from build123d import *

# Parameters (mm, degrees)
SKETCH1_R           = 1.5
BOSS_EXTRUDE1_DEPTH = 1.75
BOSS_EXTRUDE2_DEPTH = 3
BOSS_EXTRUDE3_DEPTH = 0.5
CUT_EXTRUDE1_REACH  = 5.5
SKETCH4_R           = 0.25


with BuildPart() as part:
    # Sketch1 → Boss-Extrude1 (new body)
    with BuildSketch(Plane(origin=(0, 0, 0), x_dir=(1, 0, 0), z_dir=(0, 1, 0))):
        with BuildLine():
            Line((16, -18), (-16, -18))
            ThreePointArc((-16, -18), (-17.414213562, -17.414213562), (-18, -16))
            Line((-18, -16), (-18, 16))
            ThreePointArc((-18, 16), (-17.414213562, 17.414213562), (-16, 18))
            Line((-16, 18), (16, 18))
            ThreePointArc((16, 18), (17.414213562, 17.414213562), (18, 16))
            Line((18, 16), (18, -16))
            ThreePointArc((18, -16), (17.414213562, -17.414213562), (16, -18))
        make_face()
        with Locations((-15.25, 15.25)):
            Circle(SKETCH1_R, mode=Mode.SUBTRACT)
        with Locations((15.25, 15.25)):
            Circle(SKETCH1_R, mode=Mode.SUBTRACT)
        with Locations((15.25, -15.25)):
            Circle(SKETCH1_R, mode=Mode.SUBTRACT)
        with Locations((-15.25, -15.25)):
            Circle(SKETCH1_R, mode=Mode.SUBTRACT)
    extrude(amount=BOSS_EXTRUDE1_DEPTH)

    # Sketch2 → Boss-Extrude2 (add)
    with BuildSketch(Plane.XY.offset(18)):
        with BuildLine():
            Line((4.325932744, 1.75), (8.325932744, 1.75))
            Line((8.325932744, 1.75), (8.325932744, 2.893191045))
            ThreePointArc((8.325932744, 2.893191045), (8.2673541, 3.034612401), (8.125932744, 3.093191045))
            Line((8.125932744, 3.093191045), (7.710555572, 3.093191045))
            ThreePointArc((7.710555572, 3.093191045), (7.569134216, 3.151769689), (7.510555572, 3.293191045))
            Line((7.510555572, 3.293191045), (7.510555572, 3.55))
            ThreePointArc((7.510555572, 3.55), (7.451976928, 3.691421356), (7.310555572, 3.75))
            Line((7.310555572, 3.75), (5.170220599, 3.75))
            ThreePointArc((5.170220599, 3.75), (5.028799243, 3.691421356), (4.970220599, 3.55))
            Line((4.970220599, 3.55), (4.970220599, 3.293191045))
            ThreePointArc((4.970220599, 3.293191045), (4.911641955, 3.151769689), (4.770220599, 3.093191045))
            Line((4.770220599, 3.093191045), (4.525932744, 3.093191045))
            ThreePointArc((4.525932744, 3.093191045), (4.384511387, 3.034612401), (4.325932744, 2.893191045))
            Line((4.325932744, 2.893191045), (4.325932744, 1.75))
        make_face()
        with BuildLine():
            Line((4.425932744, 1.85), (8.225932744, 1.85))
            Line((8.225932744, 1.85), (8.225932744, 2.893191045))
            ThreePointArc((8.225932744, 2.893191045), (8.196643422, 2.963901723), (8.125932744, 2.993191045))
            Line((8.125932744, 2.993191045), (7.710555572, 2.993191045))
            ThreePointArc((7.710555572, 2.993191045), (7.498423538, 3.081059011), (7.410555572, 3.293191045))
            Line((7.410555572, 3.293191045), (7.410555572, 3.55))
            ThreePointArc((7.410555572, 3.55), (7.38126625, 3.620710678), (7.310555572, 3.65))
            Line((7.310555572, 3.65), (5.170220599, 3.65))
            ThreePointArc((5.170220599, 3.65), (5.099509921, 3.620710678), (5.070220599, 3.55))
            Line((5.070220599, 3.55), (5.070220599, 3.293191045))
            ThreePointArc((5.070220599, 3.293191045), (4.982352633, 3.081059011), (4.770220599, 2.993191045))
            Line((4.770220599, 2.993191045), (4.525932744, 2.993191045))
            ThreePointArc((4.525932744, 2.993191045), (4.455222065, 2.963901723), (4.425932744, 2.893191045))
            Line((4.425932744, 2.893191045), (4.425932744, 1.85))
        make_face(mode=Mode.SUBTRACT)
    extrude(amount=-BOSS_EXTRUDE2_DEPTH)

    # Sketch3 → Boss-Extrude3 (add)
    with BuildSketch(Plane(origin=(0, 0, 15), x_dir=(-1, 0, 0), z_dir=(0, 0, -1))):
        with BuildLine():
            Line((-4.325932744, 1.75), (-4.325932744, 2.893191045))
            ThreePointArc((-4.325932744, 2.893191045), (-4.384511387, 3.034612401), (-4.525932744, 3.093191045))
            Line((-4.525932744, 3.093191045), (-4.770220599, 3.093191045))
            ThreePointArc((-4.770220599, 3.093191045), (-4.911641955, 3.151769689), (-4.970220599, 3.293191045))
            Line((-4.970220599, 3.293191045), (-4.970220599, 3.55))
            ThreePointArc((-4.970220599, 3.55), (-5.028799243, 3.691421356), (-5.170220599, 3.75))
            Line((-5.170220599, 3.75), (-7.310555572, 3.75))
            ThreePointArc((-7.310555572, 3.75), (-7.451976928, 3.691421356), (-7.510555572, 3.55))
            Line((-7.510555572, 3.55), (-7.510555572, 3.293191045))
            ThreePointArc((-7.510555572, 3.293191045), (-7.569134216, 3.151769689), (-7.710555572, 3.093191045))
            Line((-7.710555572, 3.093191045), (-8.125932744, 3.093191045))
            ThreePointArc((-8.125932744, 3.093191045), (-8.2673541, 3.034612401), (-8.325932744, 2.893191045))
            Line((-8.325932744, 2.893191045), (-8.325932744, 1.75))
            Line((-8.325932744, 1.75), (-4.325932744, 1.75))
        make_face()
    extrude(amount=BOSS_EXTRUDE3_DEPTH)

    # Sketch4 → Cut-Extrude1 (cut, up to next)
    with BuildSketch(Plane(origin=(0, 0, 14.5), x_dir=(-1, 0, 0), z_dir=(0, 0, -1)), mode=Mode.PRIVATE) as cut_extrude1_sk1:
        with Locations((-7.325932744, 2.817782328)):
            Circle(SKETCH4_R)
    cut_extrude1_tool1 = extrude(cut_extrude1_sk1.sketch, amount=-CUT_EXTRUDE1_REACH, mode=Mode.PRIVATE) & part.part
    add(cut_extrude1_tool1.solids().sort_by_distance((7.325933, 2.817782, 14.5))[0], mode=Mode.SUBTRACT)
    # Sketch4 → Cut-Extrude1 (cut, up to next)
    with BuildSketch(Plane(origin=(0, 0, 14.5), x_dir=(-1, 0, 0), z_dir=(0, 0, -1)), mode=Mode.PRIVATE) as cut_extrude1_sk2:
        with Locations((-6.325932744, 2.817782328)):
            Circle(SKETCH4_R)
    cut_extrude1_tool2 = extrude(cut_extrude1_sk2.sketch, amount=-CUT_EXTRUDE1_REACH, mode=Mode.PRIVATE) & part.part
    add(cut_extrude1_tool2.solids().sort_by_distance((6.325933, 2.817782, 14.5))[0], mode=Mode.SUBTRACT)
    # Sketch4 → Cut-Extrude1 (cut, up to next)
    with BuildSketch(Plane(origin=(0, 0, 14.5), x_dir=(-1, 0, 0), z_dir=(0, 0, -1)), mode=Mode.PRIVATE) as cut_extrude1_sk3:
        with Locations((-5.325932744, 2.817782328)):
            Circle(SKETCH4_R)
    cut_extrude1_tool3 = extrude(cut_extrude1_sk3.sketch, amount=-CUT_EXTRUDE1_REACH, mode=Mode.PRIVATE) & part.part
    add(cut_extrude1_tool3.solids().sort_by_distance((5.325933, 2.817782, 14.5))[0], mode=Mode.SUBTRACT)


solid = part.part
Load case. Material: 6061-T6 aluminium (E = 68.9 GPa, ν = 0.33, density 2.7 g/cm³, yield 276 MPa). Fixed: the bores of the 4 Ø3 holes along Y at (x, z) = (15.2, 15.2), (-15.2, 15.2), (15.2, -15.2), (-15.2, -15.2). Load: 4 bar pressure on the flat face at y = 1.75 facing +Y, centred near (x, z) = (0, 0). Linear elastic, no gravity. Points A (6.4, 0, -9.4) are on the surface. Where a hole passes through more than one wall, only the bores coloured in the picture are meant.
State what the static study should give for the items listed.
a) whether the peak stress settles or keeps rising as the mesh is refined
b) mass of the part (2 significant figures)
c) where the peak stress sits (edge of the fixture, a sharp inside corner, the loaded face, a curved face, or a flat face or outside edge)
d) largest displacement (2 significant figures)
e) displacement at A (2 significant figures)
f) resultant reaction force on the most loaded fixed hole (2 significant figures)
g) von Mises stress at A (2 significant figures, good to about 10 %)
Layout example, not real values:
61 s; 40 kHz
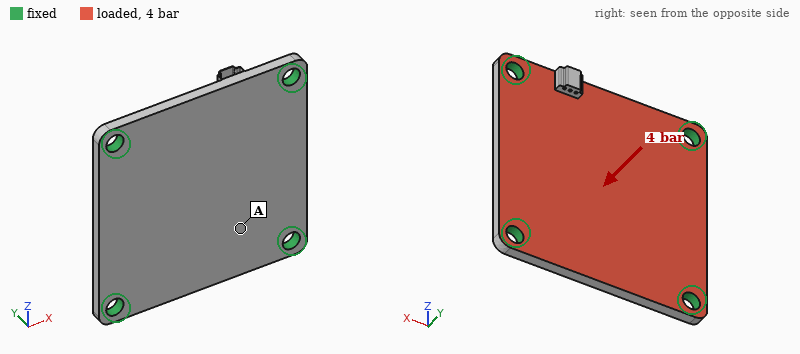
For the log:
keeps rising; 6.0 g; edge of the fixture; 65 µm; 40 µm; 130 N; 20 MPa
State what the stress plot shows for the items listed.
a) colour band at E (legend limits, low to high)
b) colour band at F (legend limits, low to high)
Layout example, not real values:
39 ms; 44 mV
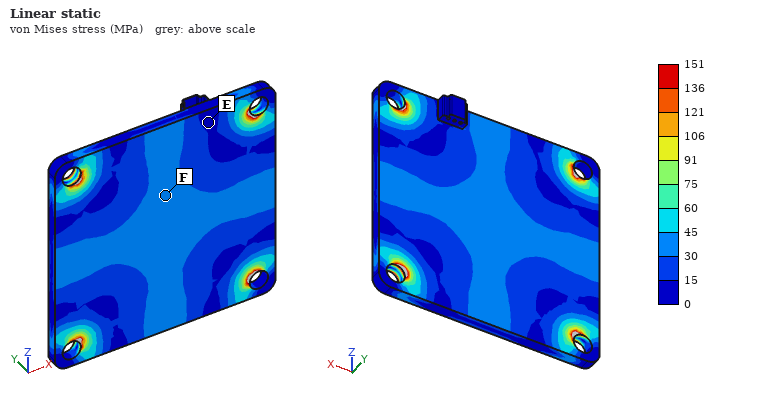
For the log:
0 to 15 MPa; 30 to 45 MPa
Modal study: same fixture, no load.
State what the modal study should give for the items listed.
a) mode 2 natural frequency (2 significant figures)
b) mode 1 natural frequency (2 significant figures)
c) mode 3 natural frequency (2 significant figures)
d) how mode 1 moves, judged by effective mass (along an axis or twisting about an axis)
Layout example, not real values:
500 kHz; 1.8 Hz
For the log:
12 kHz; 7000 Hz; 12 kHz; along Y
